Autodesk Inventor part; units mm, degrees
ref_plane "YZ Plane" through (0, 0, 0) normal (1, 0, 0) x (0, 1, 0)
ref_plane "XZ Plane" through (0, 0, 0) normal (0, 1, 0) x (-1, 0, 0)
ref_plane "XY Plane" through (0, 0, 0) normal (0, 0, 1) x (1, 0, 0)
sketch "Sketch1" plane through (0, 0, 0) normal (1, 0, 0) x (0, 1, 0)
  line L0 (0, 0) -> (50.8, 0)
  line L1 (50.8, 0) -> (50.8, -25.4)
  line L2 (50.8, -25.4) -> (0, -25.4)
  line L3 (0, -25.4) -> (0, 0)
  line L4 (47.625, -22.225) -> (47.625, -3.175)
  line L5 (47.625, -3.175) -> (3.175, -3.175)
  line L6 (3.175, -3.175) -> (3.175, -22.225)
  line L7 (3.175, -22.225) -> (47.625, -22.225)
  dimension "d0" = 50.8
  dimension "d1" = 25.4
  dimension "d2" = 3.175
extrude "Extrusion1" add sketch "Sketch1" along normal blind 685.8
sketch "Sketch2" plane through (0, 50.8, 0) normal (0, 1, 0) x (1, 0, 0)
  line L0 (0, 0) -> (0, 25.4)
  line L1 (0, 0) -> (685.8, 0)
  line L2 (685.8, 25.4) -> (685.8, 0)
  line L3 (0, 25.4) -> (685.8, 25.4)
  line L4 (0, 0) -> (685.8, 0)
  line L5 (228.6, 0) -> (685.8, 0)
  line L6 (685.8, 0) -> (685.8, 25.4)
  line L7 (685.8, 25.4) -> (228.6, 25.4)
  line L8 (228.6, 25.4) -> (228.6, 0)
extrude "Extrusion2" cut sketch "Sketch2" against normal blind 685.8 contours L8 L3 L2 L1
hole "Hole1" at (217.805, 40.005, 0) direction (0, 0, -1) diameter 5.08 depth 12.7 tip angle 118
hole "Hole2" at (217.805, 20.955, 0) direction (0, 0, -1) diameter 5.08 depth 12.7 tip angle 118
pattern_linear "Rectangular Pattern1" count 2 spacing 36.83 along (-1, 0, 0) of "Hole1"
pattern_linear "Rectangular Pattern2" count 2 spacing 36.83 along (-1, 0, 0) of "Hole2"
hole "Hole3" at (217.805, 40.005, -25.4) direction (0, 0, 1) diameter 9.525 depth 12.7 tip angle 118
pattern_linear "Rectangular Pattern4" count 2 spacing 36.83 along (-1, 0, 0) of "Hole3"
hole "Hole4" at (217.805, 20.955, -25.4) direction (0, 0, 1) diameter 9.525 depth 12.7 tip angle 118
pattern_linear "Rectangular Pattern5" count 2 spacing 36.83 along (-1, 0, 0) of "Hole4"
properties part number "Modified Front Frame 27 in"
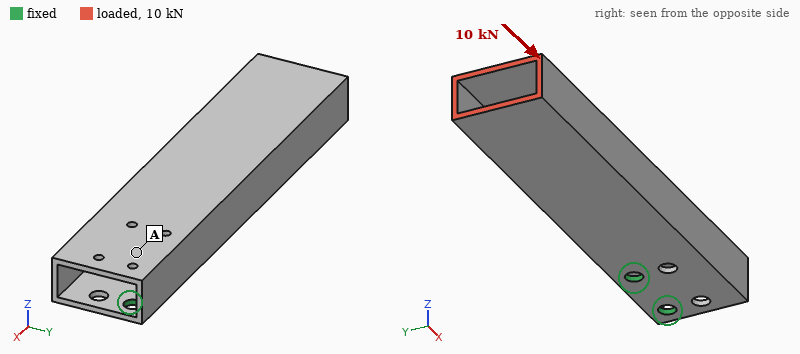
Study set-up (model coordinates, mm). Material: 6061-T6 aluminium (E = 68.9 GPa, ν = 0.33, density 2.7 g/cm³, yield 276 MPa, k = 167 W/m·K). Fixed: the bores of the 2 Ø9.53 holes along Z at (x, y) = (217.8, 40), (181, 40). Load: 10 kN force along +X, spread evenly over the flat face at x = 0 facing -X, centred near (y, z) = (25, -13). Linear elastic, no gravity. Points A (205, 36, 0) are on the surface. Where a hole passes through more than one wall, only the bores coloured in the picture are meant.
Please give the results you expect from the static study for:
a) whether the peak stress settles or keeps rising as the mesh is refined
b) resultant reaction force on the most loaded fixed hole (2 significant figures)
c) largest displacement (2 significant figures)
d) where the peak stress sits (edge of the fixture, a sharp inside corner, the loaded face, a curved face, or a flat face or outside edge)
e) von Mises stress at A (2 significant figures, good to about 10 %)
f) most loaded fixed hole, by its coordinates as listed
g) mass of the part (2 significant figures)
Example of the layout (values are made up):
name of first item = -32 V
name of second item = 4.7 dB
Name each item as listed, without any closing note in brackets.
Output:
whether the peak stress settles or keeps rising as the mesh is refined = keeps rising
resultant reaction force on the most loaded fixed hole = 7.0 kN
largest displacement = 1.1 mm
where the peak stress sits = edge of the fixture
von Mises stress at A = 38 MPa
most loaded fixed hole, by its coordinates as listed = (181, 40)
mass of the part = 270 g
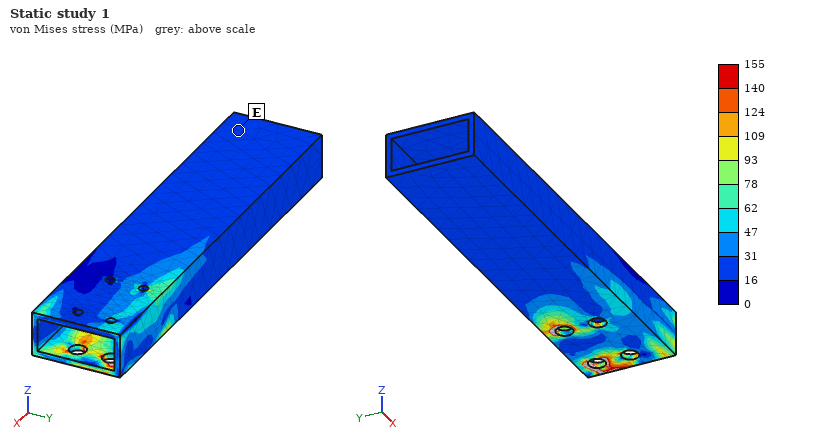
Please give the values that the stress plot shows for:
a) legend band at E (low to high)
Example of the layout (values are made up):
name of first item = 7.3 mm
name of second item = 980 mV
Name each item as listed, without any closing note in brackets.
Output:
legend band at E = 16 to 31 MPa
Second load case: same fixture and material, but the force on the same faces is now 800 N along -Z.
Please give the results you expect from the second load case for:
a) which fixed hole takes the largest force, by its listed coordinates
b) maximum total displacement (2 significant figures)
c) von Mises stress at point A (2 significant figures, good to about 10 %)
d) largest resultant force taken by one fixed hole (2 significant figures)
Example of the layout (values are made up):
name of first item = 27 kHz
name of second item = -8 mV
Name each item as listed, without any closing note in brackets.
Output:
which fixed hole takes the largest force, by its listed coordinates = (181, 40)
maximum total displacement = 2.1 mm
von Mises stress at point A = 51 MPa
largest resultant force taken by one fixed hole = 4.9 kN
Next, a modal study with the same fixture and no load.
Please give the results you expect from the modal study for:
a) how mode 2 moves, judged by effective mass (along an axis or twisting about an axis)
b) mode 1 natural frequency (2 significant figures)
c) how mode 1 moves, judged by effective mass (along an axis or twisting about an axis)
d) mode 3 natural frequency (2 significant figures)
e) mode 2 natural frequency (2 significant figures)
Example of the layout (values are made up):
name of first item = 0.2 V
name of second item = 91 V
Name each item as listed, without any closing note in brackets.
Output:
how mode 2 moves, judged by effective mass = along Y
mode 1 natural frequency = 360 Hz
how mode 1 moves, judged by effective mass = along Z
mode 3 natural frequency = 920 Hz
mode 2 natural frequency = 620 Hz
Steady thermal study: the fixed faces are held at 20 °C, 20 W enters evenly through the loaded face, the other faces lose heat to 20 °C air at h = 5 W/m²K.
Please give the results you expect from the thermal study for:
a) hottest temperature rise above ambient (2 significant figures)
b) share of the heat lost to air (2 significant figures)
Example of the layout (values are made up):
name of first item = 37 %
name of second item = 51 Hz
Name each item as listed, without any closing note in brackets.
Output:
hottest temperature rise above ambient = 45 K
share of the heat lost to air = 31 %
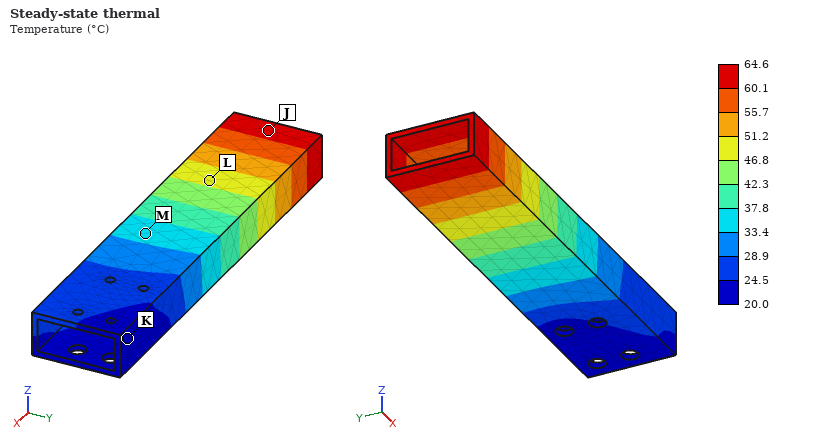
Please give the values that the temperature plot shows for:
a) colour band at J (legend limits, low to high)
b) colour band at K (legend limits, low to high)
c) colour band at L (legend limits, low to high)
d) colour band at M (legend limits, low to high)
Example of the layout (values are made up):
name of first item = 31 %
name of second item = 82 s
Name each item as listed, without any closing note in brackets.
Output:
colour band at J = 60.1 to 64.6 °C
colour band at K = 20.0 to 24.5 °C
colour band at L = 46.8 to 51.2 °C
colour band at M = 33.4 to 37.8 °C
